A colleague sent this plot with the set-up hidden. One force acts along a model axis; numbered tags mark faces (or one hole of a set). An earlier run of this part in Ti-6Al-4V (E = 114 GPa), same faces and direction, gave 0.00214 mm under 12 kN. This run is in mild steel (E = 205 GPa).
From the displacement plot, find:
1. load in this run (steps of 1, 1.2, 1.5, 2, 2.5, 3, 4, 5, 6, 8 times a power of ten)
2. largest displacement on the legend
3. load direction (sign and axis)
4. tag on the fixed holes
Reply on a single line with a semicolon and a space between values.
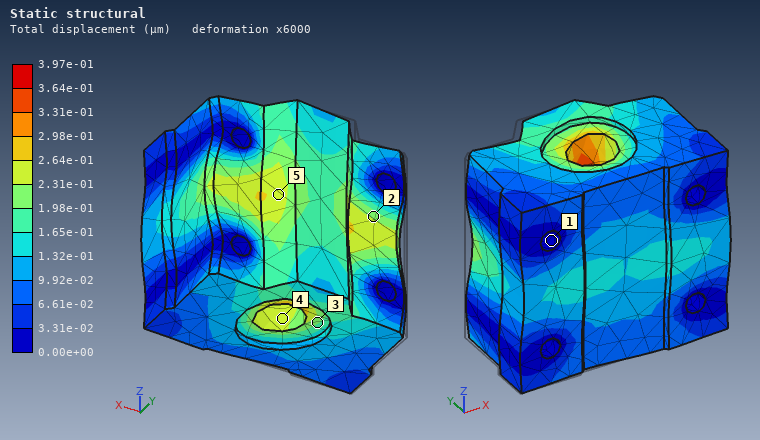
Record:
4 kN; 3.97e-01 µm; +X; 1
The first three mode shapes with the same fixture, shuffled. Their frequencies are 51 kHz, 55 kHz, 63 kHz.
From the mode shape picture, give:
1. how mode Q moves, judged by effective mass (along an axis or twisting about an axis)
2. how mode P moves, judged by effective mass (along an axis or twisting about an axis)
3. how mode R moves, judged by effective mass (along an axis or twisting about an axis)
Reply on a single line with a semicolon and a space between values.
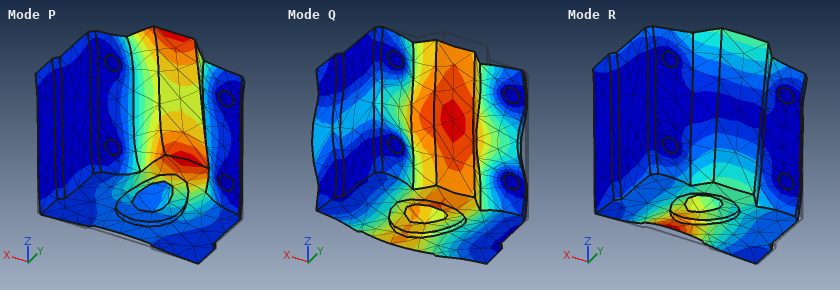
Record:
along Y; along Z; along Z
